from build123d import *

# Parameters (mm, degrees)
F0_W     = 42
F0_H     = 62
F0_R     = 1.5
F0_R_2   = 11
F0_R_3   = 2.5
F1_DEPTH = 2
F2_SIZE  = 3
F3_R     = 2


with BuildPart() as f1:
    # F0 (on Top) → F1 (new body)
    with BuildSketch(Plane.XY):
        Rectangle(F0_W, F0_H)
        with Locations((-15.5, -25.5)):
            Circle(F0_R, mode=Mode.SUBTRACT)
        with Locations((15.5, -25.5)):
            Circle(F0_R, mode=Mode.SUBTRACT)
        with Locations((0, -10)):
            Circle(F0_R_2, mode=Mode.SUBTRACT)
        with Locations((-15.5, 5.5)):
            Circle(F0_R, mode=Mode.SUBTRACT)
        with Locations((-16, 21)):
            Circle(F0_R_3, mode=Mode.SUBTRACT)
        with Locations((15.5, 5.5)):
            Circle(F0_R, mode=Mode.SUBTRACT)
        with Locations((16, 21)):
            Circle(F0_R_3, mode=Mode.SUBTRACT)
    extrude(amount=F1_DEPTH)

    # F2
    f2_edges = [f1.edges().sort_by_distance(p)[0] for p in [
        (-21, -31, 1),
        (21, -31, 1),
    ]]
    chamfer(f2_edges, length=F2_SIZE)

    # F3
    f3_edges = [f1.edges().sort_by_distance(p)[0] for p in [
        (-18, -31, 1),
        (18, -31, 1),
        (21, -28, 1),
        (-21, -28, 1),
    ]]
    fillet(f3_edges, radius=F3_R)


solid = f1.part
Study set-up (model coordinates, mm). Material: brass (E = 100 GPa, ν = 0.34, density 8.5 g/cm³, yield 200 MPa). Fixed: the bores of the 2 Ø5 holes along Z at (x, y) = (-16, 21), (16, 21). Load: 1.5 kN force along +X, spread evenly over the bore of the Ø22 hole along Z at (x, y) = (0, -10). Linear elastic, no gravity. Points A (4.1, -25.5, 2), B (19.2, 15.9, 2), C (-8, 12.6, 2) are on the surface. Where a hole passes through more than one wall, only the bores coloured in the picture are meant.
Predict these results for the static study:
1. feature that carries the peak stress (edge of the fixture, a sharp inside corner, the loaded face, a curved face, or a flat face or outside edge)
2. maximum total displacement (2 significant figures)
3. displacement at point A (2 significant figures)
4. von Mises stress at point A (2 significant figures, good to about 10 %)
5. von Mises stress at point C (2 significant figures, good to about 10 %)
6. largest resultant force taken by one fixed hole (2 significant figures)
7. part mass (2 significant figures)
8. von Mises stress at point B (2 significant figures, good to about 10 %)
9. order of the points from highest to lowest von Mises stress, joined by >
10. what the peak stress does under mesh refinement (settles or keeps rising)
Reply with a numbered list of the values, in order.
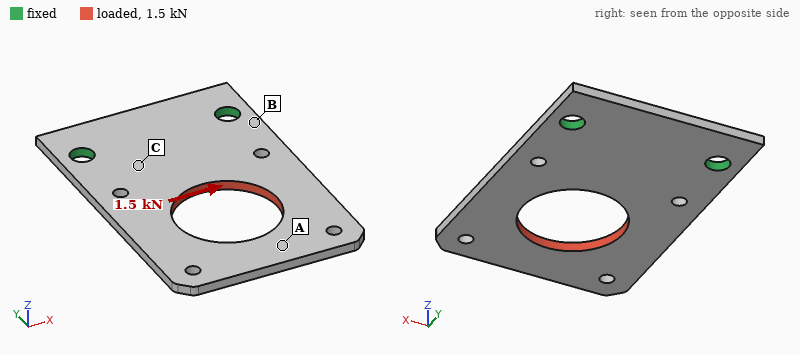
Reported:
1. edge of the fixture
2. 77 µm
3. 70 µm
4. 21 MPa
5. 43 MPa
6. 1.6 kN
7. 36 g
8. 68 MPa
9. B > C > A
10. keeps rising
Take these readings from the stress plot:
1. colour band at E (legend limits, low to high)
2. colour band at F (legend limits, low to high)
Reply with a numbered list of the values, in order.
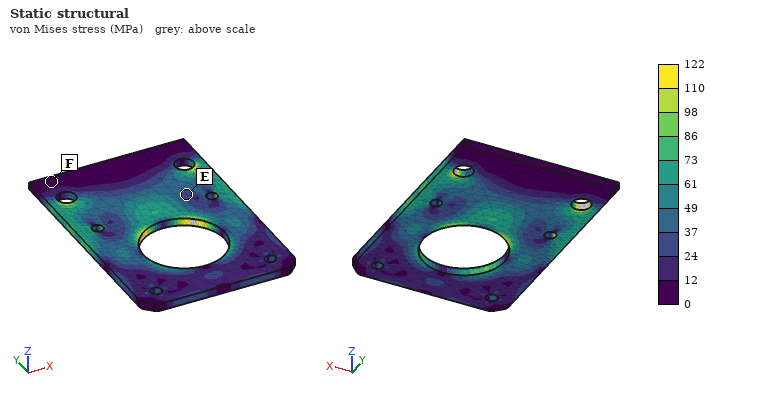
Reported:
1. 24 to 37 MPa
2. 0 to 12 MPa
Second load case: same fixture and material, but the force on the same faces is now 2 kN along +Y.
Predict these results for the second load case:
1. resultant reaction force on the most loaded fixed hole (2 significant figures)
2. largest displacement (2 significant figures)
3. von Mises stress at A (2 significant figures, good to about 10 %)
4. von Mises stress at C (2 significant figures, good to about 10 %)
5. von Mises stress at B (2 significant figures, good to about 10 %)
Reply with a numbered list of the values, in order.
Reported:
1. 1.0 kN
2. 21 µm
3. 18 MPa
4. 18 MPa
5. 37 MPa
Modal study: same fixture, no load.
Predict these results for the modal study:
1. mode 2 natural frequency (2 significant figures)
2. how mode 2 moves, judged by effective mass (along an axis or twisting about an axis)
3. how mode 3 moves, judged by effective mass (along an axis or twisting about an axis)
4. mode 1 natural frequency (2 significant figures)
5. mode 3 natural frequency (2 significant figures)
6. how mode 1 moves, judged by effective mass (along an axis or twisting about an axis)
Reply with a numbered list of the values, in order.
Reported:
1. 1100 Hz
2. twisting about Y
3. along Z
4. 430 Hz
5. 2400 Hz
6. along Z
